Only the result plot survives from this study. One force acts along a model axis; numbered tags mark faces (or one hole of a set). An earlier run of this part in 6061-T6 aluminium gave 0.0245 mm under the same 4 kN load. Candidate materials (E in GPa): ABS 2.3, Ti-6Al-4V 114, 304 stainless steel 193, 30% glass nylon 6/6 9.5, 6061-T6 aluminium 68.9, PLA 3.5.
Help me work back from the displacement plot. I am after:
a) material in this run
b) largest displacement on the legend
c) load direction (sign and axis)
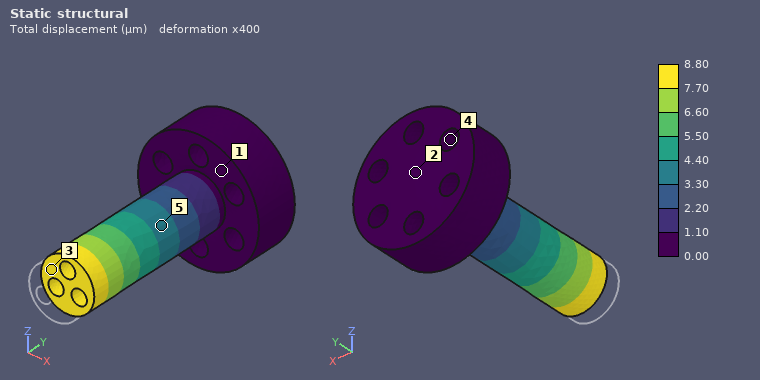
304 stainless steel
8.80 µm
+Y
